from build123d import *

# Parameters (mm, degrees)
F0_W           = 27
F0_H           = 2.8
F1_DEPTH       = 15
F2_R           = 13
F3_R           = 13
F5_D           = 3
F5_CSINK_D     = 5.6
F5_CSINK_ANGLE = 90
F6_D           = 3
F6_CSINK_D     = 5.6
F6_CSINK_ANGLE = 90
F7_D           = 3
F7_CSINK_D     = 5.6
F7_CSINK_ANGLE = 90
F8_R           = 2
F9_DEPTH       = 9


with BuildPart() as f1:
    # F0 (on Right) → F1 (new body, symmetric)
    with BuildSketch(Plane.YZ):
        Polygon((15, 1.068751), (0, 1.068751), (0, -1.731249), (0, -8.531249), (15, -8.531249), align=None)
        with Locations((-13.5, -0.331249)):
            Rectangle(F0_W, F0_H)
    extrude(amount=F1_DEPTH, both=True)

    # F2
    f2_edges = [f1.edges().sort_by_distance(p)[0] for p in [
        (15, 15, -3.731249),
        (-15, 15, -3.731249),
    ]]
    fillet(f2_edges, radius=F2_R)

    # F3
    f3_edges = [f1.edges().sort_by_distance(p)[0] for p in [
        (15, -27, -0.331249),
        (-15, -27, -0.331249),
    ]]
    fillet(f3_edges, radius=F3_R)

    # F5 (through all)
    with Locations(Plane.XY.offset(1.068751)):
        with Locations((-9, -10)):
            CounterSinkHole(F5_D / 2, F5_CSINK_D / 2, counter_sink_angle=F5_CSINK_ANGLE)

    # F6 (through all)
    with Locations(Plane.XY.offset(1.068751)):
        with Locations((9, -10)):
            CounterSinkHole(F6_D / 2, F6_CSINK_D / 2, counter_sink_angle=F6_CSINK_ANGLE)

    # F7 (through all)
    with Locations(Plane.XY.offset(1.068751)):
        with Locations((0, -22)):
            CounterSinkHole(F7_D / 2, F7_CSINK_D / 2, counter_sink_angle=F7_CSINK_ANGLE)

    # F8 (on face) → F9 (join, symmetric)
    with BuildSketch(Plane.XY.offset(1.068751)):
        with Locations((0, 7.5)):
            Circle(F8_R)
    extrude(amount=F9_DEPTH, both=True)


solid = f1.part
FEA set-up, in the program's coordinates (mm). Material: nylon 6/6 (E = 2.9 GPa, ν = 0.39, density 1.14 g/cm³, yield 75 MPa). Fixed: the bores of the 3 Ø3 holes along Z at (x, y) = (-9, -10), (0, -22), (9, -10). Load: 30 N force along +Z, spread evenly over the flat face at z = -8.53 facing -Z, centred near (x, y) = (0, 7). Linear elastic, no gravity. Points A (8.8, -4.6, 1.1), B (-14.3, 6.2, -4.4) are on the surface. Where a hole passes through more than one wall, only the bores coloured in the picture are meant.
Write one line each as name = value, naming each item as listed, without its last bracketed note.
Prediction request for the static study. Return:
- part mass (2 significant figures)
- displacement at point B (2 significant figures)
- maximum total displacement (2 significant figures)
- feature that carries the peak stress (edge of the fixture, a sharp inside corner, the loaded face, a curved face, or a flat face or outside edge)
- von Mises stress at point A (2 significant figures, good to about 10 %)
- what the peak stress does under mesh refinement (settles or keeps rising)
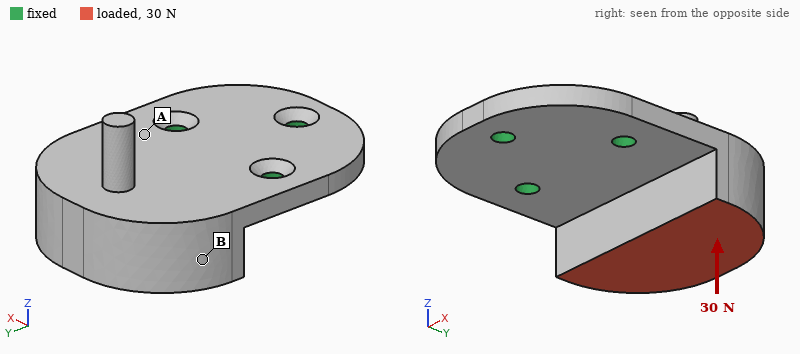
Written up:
part mass = 6.5 g
displacement at point B = 0.36 mm
maximum total displacement = 0.63 mm
feature that carries the peak stress = edge of the fixture
von Mises stress at point A = 6.8 MPa
what the peak stress does under mesh refinement = keeps rising
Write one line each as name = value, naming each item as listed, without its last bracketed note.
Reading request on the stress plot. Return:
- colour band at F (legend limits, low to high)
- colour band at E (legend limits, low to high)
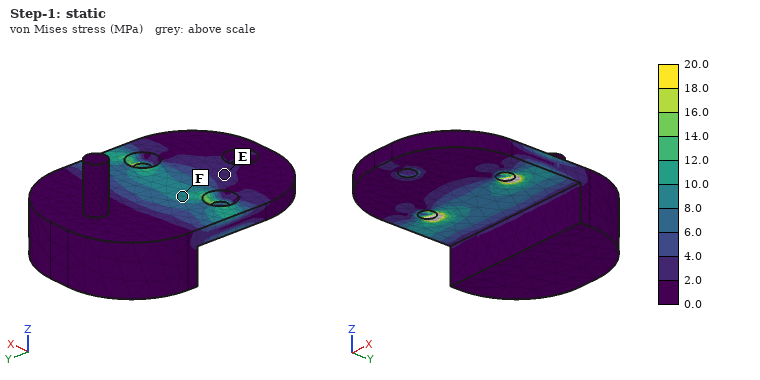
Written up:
colour band at F = 8.0 to 10.0 MPa
colour band at E = 2.0 to 4.0 MPa
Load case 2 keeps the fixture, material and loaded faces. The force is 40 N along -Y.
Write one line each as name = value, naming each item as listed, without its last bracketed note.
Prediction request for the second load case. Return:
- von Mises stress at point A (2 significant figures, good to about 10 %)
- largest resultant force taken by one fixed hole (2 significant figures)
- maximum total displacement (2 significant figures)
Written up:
von Mises stress at point A = 6.2 MPa
largest resultant force taken by one fixed hole = 26 N
maximum total displacement = 0.54 mm
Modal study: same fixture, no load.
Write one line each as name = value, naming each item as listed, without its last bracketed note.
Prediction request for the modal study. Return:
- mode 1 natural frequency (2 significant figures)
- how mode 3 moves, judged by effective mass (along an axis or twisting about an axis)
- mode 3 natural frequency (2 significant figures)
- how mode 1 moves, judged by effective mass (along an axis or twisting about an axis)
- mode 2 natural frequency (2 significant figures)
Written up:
mode 1 natural frequency = 640 Hz
how mode 3 moves, judged by effective mass = along X
mode 3 natural frequency = 4100 Hz
how mode 1 moves, judged by effective mass = along Z
mode 2 natural frequency = 2200 Hz
